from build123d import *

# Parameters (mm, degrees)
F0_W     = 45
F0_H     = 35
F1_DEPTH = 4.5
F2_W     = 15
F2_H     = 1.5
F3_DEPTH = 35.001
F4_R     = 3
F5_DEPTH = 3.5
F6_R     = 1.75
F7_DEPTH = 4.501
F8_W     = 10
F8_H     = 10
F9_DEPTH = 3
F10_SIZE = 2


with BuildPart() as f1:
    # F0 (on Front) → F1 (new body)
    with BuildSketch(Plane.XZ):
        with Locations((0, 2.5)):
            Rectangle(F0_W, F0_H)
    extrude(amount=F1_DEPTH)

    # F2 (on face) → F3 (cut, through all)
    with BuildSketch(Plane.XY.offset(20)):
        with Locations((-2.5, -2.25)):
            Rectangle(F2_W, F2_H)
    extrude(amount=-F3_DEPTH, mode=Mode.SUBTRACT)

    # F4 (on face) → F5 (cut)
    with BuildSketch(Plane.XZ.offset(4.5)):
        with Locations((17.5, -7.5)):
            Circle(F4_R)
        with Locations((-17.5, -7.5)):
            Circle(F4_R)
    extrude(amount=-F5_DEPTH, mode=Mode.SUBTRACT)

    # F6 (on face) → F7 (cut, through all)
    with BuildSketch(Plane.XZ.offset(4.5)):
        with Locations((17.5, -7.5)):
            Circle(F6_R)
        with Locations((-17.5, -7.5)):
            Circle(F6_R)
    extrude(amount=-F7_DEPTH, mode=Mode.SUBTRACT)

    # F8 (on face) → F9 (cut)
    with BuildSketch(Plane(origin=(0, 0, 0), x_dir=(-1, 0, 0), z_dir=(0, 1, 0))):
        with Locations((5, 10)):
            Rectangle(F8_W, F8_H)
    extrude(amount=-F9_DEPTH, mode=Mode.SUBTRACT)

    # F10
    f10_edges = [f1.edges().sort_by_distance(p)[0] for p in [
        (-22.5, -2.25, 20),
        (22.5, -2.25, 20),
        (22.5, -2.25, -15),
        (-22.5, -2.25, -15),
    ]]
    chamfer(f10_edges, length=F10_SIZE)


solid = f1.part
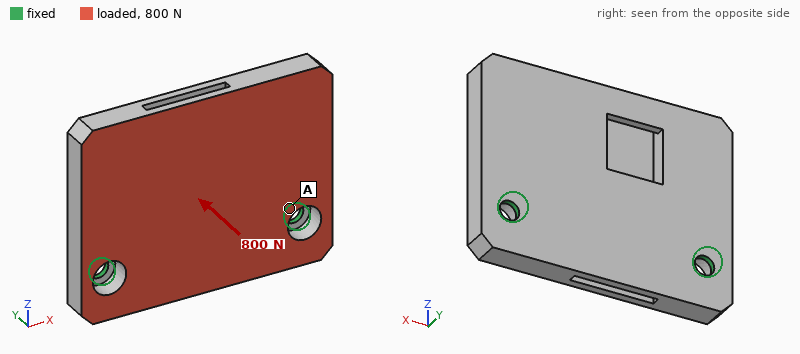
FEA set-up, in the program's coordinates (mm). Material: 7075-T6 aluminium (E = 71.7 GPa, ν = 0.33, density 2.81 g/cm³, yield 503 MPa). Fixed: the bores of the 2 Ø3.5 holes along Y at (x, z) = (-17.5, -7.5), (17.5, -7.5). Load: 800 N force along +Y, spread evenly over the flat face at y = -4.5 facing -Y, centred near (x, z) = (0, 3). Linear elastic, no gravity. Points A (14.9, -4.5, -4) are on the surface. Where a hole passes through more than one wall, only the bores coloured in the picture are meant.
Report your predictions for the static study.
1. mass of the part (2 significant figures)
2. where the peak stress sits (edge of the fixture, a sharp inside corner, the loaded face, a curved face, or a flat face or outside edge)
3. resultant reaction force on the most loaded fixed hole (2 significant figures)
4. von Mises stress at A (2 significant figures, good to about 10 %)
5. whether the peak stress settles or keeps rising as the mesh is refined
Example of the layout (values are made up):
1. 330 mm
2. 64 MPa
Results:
1. 17 g
2. edge of the fixture
3. 510 N
4. 87 MPa
5. keeps rising
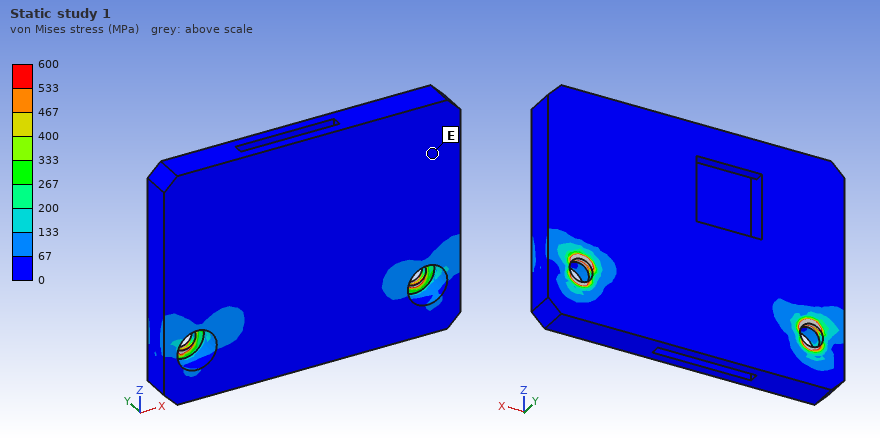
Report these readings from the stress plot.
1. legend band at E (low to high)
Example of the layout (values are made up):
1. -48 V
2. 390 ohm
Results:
1. 0 to 67 MPa
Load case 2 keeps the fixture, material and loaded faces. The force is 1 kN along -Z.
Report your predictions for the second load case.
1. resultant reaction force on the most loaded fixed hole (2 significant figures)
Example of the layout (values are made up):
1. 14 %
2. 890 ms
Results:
1. 500 N
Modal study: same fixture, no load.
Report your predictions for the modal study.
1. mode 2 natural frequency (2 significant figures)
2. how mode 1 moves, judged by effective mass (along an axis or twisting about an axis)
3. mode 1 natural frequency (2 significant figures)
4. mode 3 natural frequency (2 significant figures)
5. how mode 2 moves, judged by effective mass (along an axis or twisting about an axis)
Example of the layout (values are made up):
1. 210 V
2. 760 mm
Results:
1. 5000 Hz
2. along Y
3. 2000 Hz
4. 11 kHz
5. twisting about Z
